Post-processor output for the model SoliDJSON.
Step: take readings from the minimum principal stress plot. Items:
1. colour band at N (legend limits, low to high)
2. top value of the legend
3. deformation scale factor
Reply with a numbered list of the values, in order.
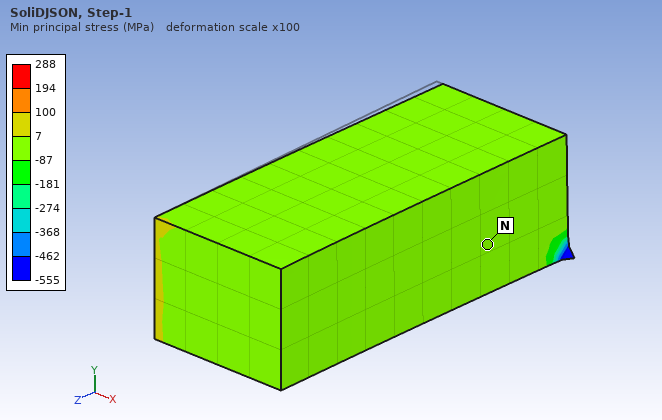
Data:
1. -87 to 7 MPa
2. 288 MPa
3. 100
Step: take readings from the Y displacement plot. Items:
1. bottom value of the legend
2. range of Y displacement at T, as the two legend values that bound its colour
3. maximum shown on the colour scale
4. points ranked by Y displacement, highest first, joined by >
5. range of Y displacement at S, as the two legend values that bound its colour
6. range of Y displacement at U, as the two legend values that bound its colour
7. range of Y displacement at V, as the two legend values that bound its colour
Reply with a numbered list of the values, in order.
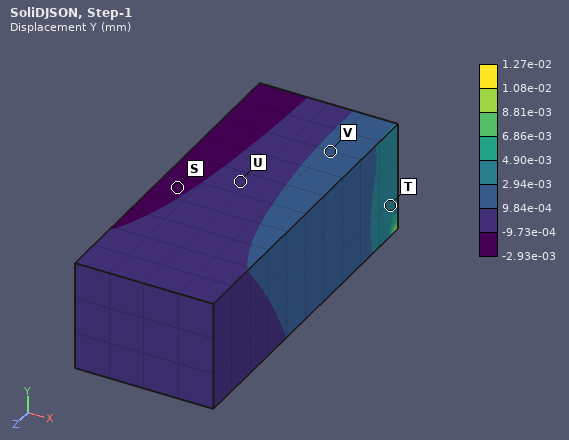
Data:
1. -2.93e-03 mm
2. 2.94e-03 to 4.90e-03 mm
3. 1.27e-02 mm
4. T > V > U > S
5. -2.93e-03 to -9.73e-04 mm
6. -9.73e-04 to 9.84e-04 mm
7. 9.84e-04 to 2.94e-03 mm
